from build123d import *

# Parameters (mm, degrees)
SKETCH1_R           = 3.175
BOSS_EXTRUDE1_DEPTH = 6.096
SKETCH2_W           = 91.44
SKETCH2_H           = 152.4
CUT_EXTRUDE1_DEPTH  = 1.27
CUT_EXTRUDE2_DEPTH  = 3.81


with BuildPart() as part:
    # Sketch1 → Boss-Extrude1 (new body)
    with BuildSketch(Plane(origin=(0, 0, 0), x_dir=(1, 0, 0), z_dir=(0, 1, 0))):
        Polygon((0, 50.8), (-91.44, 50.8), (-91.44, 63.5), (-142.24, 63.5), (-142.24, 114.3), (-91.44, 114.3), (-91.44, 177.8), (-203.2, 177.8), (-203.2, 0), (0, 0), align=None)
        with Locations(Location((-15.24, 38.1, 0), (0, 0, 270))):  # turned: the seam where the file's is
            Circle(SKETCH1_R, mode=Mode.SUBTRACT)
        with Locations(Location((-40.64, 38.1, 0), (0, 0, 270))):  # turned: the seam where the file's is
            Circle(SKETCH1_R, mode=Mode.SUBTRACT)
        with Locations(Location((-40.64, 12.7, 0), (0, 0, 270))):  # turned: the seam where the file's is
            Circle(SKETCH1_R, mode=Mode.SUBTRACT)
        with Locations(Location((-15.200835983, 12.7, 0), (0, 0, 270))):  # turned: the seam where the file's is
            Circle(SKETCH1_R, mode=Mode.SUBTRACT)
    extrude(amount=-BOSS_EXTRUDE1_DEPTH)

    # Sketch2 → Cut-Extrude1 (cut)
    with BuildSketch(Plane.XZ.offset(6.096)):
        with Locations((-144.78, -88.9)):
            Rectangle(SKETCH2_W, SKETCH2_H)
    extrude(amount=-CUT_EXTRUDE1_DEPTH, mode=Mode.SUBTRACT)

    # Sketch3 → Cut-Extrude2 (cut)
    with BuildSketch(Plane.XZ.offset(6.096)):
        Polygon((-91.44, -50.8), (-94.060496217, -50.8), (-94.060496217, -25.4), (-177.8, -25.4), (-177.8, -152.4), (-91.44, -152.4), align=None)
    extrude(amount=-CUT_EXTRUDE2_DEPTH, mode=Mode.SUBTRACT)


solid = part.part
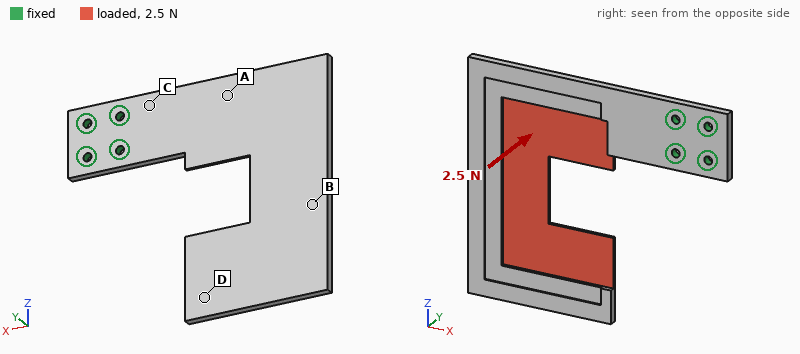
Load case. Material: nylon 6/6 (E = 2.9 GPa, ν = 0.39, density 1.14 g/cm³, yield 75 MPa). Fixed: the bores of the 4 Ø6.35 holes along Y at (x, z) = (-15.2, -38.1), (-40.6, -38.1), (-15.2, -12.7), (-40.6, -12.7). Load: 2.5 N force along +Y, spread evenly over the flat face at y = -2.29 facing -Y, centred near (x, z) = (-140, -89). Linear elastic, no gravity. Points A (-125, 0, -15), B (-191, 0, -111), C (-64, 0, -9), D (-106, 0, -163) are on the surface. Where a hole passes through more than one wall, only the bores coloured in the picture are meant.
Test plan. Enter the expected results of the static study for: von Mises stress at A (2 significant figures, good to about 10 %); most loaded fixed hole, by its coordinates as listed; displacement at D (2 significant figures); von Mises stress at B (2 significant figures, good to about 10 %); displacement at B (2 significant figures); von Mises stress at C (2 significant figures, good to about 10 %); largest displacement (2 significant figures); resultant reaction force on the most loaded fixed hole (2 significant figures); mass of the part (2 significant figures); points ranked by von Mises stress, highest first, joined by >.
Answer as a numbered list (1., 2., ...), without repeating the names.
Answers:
1. 0.93 MPa
2. (-40.6, -38.1)
3. 2.4 mm
4. 0.31 MPa
5. 1.8 mm
6. 0.72 MPa
7. 2.8 mm
8. 7.5 N
9. 110 g
10. A > C > B > D
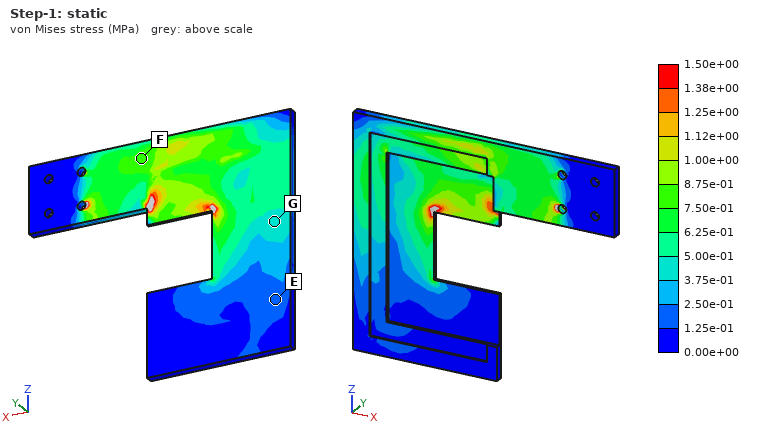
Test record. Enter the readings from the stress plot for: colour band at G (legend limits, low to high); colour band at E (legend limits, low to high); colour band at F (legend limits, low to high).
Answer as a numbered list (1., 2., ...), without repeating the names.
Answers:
1. 3.75e-01 to 5.00e-01 MPa
2. 1.25e-01 to 2.50e-01 MPa
3. 7.50e-01 to 8.75e-01 MPa
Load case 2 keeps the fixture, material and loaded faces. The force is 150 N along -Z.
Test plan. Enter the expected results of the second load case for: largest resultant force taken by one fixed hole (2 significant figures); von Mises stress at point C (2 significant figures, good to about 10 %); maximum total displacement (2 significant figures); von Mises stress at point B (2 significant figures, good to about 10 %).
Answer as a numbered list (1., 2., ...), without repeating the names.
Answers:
1. 400 N
2. 3.1 MPa
3. 2.6 mm
4. 0.97 MPa
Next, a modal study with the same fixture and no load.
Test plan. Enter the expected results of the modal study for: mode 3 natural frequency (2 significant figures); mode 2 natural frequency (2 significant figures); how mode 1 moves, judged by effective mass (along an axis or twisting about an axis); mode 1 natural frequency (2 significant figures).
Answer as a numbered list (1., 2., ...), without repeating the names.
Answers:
1. 96 Hz
2. 42 Hz
3. along Y
4. 19 Hz
